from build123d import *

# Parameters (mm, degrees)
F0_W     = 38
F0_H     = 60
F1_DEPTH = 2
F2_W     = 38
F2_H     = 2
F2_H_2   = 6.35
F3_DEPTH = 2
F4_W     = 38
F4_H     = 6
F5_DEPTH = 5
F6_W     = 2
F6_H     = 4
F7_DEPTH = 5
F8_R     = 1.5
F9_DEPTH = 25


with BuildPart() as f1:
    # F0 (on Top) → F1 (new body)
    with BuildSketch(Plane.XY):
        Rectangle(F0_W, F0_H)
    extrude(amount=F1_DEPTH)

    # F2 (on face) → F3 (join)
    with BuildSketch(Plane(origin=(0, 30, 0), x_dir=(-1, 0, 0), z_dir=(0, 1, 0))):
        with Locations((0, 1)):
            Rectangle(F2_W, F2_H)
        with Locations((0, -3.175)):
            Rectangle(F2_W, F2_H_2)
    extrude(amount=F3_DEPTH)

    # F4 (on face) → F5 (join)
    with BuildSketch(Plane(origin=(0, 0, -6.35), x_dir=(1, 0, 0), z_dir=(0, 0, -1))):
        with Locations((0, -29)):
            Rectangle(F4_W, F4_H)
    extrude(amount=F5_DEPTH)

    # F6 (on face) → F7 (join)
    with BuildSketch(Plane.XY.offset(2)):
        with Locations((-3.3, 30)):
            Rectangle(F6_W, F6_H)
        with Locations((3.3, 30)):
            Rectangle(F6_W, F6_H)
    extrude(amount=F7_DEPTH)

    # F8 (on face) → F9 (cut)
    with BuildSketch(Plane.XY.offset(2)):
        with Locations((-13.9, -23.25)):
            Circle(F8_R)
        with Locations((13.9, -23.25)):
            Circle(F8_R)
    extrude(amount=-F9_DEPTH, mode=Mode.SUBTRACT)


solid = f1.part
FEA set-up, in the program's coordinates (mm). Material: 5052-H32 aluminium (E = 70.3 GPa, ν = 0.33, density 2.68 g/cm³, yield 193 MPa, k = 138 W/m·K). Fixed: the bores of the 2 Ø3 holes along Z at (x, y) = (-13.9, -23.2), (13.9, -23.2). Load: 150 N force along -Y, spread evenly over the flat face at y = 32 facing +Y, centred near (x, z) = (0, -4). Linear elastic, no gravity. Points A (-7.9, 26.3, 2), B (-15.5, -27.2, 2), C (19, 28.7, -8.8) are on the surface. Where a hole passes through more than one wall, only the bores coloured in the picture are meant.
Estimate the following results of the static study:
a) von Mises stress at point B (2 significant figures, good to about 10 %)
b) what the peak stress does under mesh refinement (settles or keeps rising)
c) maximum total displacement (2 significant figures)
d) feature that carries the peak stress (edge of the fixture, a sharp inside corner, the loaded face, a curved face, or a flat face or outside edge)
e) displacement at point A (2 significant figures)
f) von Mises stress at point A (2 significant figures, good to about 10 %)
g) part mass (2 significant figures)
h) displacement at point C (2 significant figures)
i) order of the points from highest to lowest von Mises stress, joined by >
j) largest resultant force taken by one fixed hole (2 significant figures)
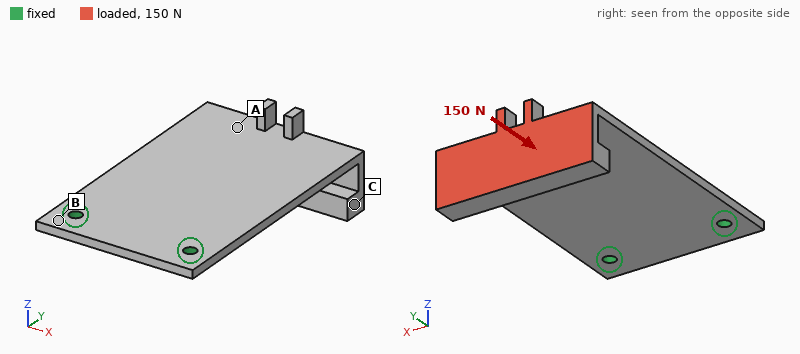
11 MPa
keeps rising
0.76 mm
edge of the fixture
0.56 mm
27 MPa
17 g
0.66 mm
A > B > C
76 N
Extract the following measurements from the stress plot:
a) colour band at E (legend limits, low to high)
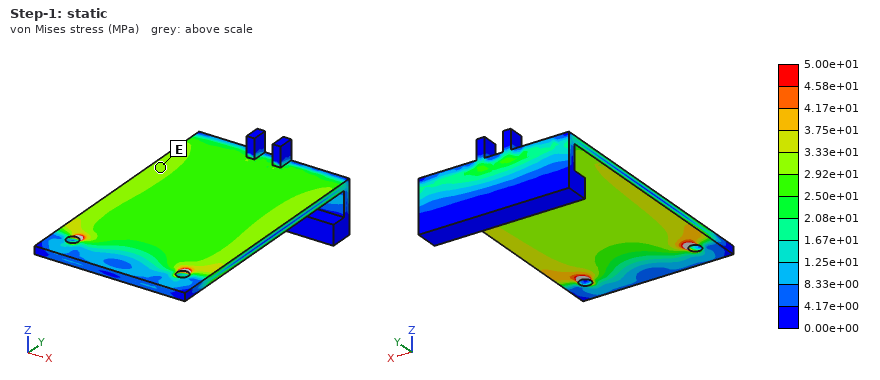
2.92e+01 to 3.33e+01 MPa
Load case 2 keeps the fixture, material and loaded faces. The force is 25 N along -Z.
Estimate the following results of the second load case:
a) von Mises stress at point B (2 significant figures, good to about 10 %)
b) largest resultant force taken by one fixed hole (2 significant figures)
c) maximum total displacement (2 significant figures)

16 MPa
13 N
0.85 mm
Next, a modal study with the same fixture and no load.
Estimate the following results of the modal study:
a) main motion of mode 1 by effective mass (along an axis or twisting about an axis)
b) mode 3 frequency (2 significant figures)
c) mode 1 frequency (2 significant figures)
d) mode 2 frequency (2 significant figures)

along Z
2100 Hz
330 Hz
1100 Hz
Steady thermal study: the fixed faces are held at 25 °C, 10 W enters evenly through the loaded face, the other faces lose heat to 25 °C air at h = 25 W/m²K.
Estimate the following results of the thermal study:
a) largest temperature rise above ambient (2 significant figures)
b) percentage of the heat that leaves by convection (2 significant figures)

44 K
33 %
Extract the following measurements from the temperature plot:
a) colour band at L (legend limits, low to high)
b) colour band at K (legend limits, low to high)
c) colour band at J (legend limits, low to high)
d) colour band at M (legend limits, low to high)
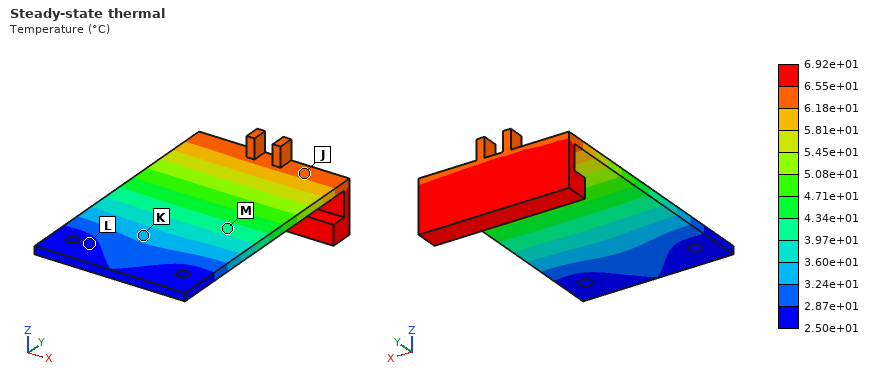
2.50e+01 to 2.87e+01 °C
3.24e+01 to 3.60e+01 °C
6.18e+01 to 6.55e+01 °C
3.97e+01 to 4.34e+01 °C
